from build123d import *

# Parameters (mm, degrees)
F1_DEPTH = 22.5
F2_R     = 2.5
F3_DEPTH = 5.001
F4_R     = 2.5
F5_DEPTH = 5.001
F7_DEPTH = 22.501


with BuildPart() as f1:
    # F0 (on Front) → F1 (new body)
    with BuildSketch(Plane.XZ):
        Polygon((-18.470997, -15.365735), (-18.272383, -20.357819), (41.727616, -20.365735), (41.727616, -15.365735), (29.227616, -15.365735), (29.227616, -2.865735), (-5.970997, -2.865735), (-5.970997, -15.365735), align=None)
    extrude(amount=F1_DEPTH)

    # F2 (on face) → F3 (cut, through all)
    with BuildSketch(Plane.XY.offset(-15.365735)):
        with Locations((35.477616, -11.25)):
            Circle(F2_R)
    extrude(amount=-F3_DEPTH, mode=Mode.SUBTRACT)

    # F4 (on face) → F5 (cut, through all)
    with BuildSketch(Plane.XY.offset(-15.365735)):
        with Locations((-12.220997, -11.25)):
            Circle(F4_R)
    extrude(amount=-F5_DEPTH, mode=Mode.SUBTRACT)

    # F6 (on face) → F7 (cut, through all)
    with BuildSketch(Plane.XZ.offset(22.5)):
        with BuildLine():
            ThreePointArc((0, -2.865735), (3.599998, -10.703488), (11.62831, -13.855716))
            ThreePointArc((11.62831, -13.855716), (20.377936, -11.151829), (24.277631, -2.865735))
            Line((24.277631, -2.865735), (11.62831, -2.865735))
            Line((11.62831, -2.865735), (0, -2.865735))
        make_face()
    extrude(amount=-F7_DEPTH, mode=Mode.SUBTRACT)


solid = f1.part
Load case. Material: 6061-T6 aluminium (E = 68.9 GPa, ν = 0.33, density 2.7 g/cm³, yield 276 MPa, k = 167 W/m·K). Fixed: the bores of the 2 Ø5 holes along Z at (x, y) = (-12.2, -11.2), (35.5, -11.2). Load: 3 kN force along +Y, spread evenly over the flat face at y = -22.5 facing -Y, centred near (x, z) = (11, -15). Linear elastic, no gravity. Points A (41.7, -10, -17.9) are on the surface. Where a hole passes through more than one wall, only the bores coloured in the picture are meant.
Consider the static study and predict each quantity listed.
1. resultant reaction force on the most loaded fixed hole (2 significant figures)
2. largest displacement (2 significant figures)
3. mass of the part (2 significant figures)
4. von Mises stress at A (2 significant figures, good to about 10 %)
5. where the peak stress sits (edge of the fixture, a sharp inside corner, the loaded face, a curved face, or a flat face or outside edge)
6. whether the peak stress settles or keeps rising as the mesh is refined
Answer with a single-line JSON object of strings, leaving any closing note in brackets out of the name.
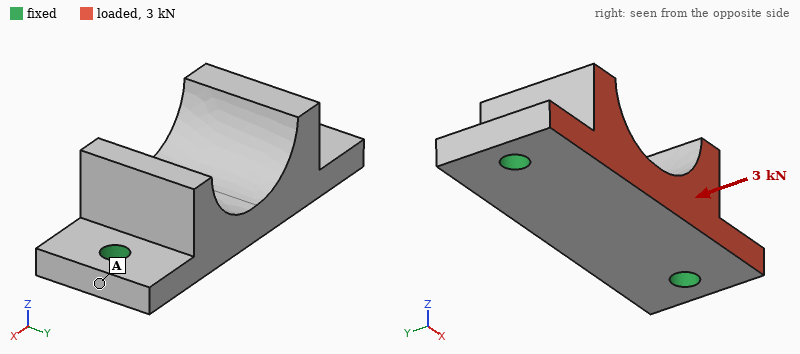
{"resultant reaction force on the most loaded fixed hole": "1.5 kN", "largest displacement": "34 µm", "mass of the part": "32 g", "von Mises stress at A": "18 MPa", "where the peak stress sits": "edge of the fixture", "whether the peak stress settles or keeps rising as the mesh is refined": "keeps rising"}
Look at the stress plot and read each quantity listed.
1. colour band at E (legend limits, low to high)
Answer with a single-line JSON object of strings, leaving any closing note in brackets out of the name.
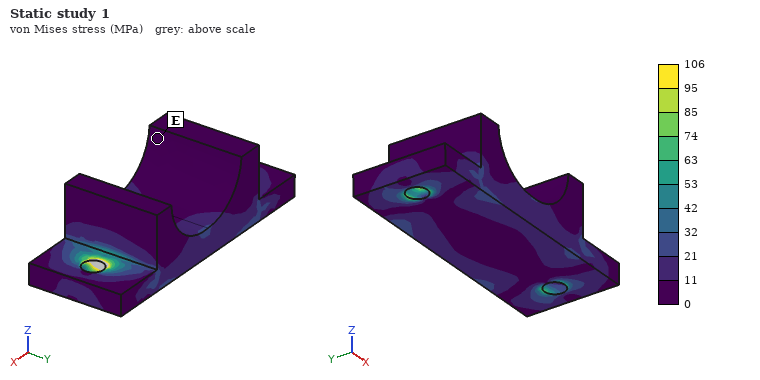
{"colour band at E": "0 to 11 MPa"}
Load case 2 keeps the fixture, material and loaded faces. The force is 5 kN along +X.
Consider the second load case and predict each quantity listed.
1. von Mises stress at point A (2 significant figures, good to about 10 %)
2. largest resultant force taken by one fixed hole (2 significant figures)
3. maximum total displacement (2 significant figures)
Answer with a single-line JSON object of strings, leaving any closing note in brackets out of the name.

{"von Mises stress at point A": "29 MPa", "largest resultant force taken by one fixed hole": "2.8 kN", "maximum total displacement": "21 µm"}
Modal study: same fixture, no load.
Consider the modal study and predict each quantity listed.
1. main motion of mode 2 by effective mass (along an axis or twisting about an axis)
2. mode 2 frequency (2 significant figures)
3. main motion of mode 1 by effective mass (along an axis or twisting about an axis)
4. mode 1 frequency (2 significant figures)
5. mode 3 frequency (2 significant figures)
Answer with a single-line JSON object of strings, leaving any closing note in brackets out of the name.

{"main motion of mode 2 by effective mass": "along Z", "mode 2 frequency": "9600 Hz", "main motion of mode 1 by effective mass": "along Y", "mode 1 frequency": "9000 Hz", "mode 3 frequency": "18 kHz"}
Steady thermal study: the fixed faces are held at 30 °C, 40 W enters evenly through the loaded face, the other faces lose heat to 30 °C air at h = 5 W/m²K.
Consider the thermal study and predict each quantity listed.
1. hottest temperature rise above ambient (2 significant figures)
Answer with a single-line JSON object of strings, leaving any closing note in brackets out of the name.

{"hottest temperature rise above ambient": "14 K"}
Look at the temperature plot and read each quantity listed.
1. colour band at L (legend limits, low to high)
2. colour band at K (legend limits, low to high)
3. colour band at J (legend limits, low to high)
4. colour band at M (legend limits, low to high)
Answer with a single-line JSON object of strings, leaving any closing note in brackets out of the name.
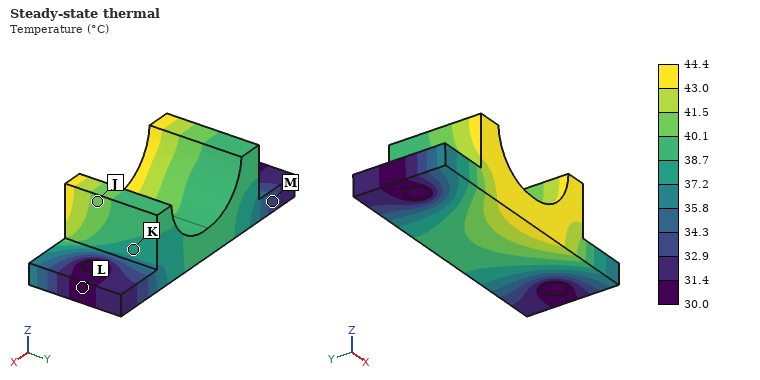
{"colour band at L": "30.0 to 31.4 °C", "colour band at K": "37.2 to 38.7 °C", "colour band at J": "40.1 to 41.5 °C", "colour band at M": "32.9 to 34.3 °C"}
